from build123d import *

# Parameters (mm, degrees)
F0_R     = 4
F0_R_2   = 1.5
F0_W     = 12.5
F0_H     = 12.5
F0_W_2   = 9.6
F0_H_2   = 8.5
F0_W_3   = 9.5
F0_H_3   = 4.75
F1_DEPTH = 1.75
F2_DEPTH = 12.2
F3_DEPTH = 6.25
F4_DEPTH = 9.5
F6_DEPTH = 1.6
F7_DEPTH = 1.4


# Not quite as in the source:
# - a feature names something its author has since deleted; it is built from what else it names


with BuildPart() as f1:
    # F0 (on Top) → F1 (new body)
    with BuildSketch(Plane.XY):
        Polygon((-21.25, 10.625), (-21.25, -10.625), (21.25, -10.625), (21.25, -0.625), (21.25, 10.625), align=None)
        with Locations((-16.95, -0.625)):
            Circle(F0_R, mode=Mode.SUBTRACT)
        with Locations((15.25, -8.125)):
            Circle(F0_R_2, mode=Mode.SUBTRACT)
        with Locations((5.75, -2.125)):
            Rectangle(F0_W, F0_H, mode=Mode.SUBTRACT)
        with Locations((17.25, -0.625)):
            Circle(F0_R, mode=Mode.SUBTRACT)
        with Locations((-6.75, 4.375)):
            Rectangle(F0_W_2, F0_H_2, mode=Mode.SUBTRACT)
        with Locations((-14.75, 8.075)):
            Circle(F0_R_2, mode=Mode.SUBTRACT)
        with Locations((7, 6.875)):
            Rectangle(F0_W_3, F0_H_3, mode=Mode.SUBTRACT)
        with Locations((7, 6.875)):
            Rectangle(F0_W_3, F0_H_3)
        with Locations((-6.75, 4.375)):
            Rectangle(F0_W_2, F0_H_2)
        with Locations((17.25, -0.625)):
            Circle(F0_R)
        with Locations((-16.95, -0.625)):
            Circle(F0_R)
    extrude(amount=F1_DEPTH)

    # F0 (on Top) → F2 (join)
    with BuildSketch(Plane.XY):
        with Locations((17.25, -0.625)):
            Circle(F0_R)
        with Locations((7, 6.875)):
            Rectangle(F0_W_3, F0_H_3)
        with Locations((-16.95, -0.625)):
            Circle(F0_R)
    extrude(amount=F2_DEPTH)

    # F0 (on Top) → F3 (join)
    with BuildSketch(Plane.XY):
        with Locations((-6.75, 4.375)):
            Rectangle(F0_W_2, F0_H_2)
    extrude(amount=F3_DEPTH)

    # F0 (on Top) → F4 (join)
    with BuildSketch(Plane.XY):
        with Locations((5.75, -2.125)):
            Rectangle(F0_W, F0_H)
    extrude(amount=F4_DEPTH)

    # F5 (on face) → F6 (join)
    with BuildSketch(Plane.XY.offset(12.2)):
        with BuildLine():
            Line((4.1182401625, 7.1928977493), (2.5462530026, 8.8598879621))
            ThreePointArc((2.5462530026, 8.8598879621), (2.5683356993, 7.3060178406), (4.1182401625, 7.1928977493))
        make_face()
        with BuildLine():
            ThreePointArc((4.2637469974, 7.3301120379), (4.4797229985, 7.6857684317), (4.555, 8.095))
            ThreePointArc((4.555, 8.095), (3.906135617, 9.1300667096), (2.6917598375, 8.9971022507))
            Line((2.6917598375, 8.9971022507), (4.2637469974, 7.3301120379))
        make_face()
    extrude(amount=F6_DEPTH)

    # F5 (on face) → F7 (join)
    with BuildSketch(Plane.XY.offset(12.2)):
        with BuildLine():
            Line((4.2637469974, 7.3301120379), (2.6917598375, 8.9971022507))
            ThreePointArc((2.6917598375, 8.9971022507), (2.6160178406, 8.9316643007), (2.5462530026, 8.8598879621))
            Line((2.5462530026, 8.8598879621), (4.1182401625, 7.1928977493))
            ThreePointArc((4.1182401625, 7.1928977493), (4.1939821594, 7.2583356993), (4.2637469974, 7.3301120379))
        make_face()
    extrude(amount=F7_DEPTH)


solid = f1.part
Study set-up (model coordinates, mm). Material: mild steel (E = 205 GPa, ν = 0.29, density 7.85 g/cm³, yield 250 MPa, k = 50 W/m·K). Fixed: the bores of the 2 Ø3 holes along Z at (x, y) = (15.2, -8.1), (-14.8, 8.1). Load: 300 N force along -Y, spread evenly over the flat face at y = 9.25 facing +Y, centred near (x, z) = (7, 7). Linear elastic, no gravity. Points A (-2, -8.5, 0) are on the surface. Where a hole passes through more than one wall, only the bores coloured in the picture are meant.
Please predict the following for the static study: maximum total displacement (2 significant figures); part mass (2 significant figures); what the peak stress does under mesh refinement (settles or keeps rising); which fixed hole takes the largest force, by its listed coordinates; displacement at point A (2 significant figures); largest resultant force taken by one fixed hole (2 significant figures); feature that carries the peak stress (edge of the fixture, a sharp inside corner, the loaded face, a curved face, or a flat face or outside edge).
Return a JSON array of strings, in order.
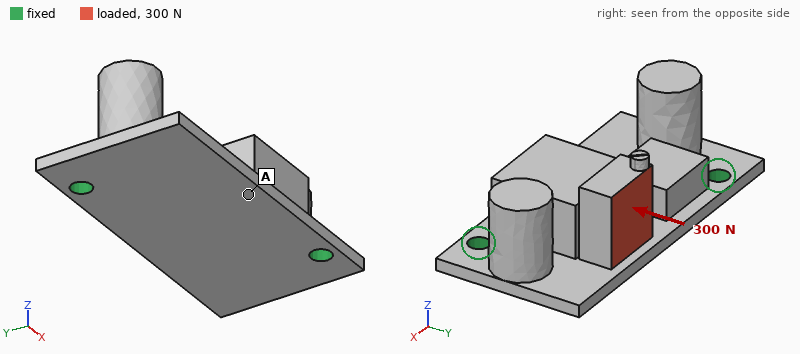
["55 µm", "37 g", "keeps rising", "(15.2, -8.1)", "12 µm", "210 N", "edge of the fixture"]
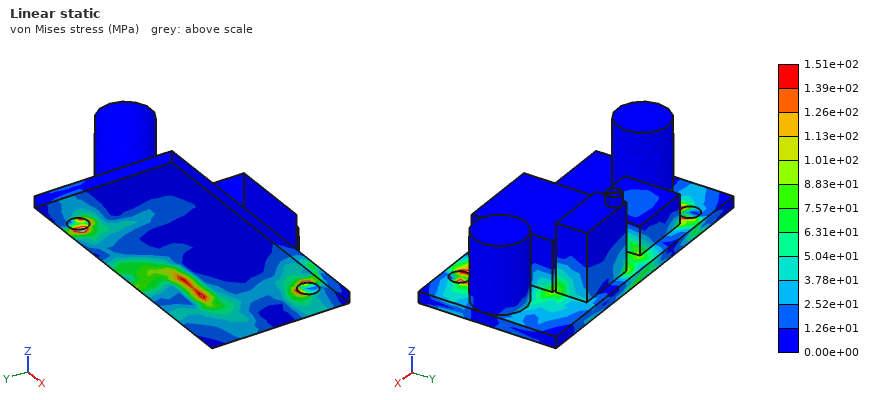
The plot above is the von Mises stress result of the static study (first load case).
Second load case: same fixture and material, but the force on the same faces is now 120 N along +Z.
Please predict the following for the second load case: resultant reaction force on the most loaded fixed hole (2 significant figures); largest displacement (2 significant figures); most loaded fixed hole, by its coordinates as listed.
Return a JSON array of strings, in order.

["80 N", "35 µm", "(15.2, -8.1)"]
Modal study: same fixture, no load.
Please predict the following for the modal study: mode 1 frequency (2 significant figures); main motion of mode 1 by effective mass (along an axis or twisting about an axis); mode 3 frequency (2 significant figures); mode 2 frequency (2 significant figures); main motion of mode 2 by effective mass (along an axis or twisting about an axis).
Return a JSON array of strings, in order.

["3200 Hz", "along Y", "5600 Hz", "4700 Hz", "along Z"]
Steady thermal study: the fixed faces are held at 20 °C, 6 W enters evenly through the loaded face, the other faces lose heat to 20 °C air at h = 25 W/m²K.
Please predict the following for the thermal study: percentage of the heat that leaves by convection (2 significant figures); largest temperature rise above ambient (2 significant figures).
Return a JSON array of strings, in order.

["19 %", "45 K"]
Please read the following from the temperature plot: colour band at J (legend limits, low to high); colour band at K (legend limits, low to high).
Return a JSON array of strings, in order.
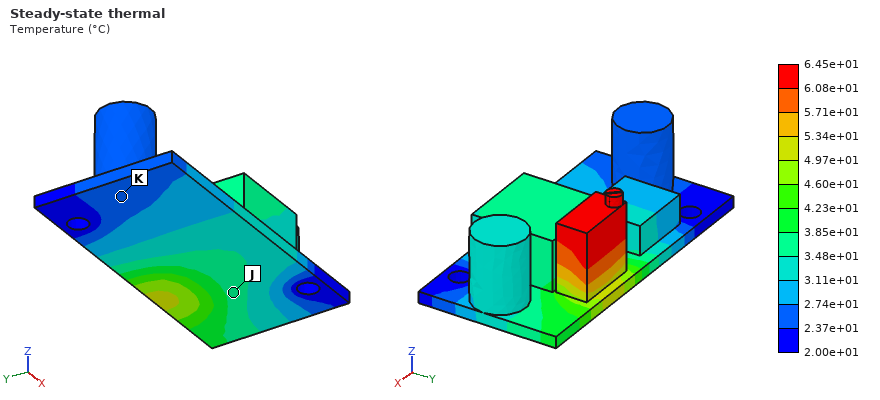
["3.48e+01 to 3.85e+01 °C", "2.37e+01 to 2.74e+01 °C"]
